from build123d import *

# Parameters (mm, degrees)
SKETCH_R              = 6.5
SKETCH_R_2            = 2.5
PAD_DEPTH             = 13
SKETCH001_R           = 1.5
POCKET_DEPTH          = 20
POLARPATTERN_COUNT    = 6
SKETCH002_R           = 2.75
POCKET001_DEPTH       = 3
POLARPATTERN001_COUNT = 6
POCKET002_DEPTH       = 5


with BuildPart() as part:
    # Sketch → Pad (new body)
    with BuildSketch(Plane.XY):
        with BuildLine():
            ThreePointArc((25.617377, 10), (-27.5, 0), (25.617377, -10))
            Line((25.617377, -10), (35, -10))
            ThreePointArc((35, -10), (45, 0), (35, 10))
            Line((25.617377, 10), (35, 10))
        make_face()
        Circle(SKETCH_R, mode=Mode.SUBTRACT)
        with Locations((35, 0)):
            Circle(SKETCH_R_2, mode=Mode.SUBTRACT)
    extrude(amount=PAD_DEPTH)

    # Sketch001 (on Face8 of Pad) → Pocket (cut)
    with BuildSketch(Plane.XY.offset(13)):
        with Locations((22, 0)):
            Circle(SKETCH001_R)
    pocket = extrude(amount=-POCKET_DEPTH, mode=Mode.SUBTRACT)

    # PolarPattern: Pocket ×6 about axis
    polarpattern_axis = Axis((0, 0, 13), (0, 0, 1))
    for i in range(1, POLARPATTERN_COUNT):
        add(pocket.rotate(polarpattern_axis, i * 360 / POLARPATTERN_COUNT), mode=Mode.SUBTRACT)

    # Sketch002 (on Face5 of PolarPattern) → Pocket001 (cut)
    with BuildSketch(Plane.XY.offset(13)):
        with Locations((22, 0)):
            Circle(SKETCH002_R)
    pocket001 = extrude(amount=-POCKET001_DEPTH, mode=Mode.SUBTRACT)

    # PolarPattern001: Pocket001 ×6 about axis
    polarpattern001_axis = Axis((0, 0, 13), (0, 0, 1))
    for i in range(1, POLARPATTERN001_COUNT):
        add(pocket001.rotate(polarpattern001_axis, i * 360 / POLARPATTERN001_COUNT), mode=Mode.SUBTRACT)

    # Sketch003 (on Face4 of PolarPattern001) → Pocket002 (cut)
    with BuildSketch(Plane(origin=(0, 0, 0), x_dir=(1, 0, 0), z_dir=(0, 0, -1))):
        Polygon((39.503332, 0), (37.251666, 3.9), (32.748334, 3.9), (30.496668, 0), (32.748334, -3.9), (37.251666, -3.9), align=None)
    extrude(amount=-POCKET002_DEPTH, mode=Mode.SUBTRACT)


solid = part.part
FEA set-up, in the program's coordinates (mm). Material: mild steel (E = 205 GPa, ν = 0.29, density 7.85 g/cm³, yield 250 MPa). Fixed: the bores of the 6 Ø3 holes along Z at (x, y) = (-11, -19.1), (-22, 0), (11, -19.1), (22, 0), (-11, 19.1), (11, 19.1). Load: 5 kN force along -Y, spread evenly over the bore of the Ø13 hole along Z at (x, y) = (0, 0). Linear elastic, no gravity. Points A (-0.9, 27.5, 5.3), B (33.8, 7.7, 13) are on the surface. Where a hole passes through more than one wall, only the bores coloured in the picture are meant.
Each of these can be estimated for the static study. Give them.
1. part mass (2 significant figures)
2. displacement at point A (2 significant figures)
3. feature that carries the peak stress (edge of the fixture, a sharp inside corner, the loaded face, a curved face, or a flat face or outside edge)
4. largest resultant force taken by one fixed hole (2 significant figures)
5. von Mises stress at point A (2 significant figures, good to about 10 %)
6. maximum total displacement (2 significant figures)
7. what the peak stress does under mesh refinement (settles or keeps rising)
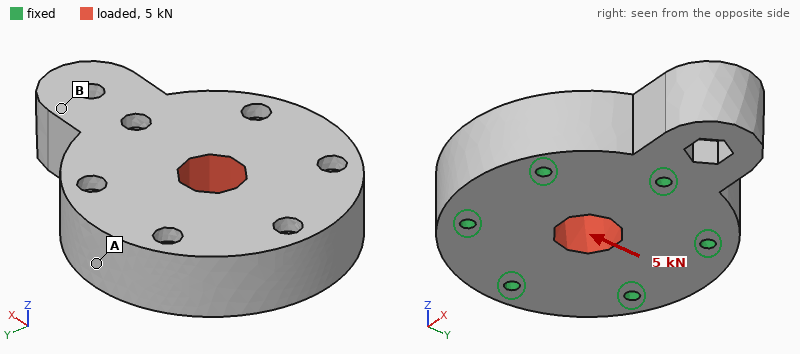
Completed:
250 g
0.33 µm
edge of the fixture
1.1 kN
4.3 MPa
0.83 µm
keeps rising
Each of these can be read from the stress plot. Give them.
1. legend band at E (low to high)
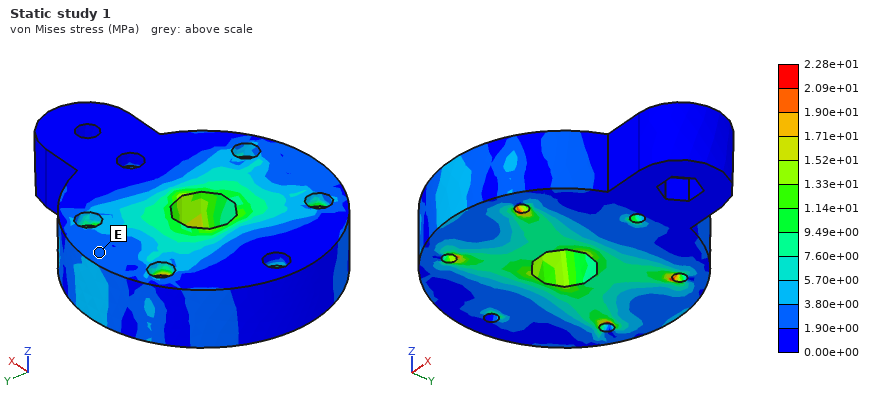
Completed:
1.90e+00 to 3.80e+00 MPa
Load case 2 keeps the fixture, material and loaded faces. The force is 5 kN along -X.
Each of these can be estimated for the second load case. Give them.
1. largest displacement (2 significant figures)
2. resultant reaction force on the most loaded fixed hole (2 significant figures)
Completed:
0.82 µm
1.3 kN
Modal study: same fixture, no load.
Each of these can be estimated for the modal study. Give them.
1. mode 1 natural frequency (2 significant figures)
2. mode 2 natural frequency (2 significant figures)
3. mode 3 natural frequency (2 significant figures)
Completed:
16 kHz
22 kHz
29 kHz
